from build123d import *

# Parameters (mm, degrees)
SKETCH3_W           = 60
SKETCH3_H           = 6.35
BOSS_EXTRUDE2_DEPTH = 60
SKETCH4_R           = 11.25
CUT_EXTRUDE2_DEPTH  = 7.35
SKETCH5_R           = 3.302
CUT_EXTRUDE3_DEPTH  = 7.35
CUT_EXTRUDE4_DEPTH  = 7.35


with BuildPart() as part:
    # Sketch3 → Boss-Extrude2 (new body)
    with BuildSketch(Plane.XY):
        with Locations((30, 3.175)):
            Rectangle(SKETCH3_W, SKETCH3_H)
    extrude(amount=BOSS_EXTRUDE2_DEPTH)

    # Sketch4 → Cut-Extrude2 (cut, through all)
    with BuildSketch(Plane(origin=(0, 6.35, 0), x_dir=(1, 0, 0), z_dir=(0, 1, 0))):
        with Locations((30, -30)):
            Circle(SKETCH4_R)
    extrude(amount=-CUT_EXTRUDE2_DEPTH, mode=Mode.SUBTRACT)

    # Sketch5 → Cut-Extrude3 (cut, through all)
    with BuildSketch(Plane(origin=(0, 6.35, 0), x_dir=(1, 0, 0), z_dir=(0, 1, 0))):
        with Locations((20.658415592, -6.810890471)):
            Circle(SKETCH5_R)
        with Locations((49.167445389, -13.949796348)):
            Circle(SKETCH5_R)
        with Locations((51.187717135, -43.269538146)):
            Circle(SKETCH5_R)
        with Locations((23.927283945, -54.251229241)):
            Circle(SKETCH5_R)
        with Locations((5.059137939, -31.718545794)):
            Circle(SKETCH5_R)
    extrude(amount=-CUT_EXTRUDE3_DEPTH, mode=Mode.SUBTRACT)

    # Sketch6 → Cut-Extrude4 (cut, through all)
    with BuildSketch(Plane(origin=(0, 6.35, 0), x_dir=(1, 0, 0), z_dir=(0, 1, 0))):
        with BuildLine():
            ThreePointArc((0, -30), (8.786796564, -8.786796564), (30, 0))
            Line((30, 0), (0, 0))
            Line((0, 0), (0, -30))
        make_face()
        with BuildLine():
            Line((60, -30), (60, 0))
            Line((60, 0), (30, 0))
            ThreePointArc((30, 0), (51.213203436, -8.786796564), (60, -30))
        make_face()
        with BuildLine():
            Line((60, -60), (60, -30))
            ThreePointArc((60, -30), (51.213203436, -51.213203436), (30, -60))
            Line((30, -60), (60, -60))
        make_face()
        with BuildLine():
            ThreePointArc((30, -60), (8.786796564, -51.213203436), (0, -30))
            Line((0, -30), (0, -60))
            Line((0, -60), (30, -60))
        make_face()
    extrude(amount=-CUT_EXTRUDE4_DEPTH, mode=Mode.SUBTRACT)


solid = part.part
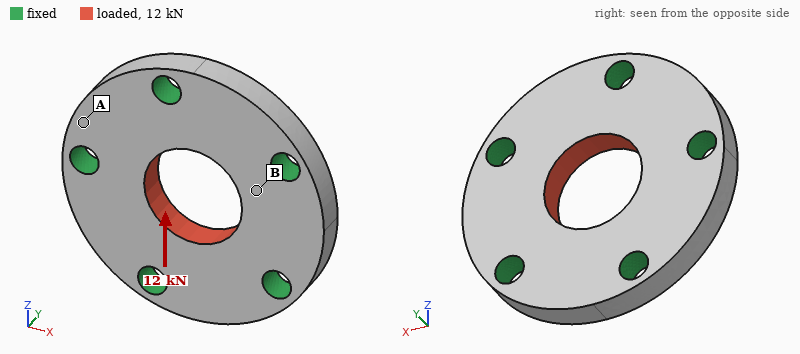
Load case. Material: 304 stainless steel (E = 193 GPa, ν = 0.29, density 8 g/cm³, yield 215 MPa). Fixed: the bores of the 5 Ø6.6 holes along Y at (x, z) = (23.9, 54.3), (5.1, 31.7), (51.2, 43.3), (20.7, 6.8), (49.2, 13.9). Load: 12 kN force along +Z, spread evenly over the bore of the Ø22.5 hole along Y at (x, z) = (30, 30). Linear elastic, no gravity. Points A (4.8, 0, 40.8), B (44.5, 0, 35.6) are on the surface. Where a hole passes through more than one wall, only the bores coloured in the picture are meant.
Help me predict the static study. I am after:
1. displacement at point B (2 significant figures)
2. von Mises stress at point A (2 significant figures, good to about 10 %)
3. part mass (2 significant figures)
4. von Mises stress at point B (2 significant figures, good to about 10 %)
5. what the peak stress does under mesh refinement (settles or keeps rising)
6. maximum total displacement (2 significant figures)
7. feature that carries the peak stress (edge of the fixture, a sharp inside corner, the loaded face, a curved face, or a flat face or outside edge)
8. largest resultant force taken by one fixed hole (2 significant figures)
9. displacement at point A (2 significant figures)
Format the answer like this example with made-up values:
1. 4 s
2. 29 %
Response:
1. 1.3 µm
2. 8.7 MPa
3. 110 g
4. 27 MPa
5. keeps rising
6. 2.8 µm
7. edge of the fixture
8. 3.2 kN
9. 0.55 µm
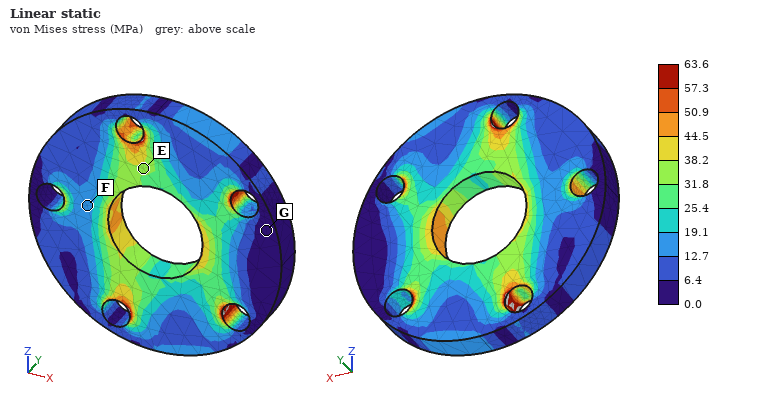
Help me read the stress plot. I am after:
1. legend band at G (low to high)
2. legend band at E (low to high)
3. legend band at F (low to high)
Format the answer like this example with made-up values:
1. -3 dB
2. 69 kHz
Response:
1. 0.0 to 6.4 MPa
2. 31.8 to 38.2 MPa
3. 12.7 to 19.1 MPa
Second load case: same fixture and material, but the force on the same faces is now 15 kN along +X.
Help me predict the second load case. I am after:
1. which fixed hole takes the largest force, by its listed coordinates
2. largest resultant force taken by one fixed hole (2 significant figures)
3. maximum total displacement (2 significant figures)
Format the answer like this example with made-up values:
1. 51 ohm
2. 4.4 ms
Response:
1. (5.1, 31.7)
2. 4.1 kN
3. 3.5 µm
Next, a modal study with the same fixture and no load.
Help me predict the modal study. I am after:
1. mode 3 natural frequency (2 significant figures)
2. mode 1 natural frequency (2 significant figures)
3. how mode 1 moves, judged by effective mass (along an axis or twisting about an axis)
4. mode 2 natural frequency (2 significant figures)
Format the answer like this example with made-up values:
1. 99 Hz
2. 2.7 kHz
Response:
1. 33 kHz
2. 29 kHz
3. along Y
4. 32 kHz
